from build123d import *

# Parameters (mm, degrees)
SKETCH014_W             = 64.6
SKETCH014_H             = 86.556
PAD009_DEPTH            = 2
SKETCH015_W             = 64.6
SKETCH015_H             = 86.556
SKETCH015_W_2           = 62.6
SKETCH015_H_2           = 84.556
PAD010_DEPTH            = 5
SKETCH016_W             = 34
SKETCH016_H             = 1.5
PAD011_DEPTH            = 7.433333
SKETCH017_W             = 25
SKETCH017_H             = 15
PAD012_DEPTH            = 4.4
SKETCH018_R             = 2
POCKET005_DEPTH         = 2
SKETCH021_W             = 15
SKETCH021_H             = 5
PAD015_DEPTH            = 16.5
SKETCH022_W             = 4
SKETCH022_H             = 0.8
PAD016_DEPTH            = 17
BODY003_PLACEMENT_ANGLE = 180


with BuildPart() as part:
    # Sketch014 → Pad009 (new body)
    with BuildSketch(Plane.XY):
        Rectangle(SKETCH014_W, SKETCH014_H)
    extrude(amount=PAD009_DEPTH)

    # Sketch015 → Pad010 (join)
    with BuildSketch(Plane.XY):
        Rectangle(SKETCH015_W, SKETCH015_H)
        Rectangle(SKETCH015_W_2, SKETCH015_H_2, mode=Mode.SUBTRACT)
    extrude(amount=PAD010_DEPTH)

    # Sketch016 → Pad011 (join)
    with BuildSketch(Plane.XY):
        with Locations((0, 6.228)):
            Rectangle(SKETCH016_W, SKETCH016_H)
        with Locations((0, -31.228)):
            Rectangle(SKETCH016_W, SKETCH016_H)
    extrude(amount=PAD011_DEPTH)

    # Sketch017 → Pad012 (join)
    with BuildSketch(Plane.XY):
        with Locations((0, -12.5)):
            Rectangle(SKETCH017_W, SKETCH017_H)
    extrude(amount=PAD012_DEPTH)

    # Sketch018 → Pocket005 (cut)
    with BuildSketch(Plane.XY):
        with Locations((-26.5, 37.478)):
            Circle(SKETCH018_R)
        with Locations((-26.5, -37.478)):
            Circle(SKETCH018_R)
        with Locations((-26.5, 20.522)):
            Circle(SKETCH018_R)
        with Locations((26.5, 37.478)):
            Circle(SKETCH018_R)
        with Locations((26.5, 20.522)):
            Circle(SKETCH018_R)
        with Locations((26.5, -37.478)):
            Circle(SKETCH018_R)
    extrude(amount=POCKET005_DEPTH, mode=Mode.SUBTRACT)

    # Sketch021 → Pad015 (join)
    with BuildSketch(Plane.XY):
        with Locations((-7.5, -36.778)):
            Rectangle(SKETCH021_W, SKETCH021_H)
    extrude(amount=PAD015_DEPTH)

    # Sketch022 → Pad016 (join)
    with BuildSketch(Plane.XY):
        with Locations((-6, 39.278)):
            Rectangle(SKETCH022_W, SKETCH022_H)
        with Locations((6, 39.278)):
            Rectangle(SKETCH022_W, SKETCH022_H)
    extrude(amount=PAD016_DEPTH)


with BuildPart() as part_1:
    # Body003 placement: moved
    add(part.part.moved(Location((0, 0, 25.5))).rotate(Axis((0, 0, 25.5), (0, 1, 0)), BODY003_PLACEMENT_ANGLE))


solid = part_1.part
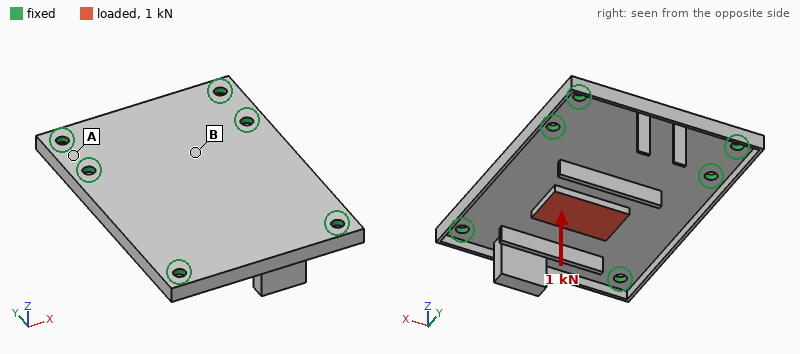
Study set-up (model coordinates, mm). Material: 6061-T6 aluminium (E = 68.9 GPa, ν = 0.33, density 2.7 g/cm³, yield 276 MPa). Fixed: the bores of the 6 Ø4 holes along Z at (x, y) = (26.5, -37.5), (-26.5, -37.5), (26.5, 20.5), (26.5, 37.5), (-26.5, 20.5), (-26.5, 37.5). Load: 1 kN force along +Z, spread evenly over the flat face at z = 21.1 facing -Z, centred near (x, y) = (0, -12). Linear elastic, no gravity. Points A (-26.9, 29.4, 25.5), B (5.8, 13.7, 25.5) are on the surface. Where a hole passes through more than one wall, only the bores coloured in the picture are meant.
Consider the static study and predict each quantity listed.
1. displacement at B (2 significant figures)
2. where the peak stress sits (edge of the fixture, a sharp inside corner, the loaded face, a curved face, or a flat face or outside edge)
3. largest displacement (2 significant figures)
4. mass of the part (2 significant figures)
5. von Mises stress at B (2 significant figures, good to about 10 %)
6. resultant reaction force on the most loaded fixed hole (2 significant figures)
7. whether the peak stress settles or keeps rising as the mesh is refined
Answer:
0.12 mm
edge of the fixture
0.31 mm
39 g
33 MPa
360 N
keeps rising
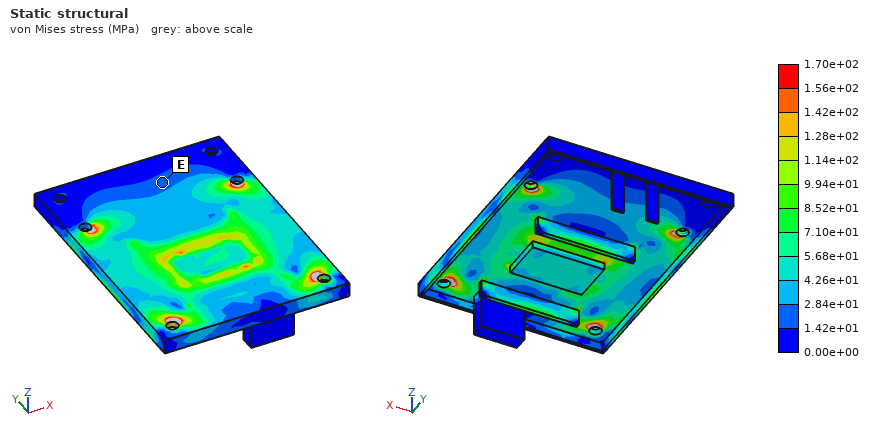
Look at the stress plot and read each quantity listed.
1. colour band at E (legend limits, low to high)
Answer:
1.42e+01 to 2.84e+01 MPa
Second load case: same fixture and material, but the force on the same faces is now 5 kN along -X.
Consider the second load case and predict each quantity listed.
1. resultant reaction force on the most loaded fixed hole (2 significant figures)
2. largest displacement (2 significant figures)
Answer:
1.6 kN
0.16 mm
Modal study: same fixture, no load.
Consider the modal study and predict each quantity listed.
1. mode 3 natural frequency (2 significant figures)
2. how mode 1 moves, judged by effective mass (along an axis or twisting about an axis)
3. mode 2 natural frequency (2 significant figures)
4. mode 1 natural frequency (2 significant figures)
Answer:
2900 Hz
along Z
2800 Hz
2700 Hz
